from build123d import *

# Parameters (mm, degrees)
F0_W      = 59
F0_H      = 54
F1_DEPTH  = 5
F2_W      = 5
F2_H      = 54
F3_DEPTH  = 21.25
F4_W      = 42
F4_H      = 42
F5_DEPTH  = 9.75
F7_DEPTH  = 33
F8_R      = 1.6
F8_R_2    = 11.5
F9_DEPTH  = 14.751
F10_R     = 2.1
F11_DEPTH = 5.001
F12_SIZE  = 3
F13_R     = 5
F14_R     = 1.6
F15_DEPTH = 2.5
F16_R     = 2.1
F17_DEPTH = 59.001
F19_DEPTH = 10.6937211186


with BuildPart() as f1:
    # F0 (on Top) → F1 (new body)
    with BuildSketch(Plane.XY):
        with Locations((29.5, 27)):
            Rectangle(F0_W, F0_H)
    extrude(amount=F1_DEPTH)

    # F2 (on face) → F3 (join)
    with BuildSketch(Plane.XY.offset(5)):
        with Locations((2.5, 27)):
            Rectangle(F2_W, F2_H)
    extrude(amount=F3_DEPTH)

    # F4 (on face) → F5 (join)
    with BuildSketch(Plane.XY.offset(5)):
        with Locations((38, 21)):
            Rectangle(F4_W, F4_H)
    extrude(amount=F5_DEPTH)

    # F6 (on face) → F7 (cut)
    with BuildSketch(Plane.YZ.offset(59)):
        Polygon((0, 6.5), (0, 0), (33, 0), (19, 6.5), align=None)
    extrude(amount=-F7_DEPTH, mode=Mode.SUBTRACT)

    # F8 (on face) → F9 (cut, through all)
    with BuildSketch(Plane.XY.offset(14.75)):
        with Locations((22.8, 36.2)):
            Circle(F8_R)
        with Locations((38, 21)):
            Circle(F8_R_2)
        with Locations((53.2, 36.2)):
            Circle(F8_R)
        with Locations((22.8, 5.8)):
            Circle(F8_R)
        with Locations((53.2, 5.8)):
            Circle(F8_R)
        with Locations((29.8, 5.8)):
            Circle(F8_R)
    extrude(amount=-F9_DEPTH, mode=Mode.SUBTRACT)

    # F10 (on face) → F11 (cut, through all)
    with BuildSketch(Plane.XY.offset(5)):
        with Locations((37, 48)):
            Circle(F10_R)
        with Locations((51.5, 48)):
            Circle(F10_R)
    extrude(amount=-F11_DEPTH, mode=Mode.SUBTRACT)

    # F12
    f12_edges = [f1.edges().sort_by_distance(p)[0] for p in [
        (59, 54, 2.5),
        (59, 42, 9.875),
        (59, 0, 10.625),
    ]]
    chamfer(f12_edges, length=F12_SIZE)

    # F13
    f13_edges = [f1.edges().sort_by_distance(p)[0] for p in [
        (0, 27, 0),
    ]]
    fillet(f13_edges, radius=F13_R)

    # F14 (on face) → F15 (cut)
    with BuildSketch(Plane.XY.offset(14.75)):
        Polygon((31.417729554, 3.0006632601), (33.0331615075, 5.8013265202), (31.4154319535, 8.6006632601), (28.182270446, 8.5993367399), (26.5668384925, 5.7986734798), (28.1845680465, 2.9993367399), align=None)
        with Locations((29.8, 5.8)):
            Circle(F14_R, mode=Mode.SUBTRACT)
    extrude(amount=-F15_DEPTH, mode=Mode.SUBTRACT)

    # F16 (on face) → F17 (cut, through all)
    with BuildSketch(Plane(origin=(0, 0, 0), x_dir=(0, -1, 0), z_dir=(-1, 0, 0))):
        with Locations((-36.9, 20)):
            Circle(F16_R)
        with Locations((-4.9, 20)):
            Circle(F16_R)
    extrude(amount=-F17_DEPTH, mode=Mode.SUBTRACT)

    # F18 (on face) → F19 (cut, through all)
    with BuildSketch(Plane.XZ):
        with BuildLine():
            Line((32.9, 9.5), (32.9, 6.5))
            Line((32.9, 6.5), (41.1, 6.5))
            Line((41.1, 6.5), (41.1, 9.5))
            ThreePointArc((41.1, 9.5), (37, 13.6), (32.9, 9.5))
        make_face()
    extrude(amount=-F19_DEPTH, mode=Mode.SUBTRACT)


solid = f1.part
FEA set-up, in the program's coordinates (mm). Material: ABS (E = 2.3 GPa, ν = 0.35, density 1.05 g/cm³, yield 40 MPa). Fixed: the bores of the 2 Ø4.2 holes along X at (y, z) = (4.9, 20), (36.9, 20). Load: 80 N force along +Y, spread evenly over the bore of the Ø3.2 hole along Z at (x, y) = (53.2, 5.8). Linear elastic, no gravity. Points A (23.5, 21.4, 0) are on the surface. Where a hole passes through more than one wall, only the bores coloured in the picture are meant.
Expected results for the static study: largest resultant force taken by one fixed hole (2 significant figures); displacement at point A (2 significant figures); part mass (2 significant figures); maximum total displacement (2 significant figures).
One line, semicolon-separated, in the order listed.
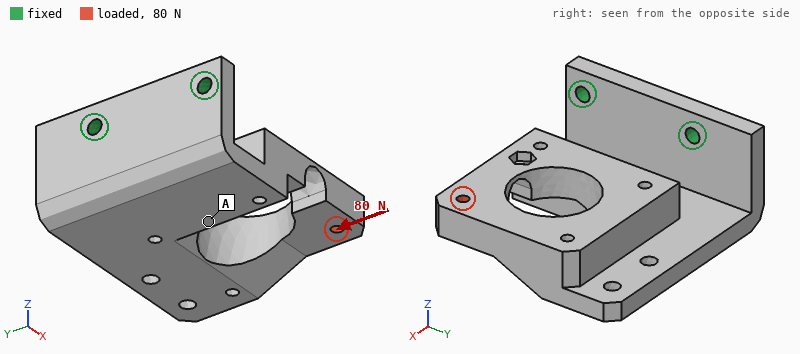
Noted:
120 N; 0.27 mm; 29 g; 0.96 mm
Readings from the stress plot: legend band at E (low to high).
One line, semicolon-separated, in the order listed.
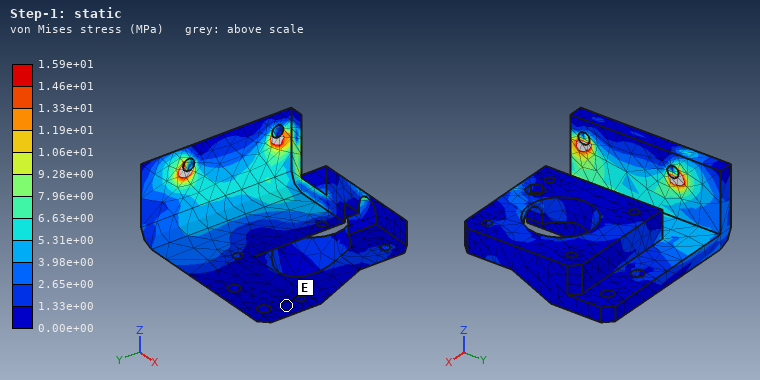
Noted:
0.00e+00 to 1.33e+00 MPa
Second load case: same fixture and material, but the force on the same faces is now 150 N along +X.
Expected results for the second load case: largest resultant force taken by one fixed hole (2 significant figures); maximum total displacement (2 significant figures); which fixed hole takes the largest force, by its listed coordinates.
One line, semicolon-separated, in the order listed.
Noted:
140 N; 0.84 mm; (4.9, 20)
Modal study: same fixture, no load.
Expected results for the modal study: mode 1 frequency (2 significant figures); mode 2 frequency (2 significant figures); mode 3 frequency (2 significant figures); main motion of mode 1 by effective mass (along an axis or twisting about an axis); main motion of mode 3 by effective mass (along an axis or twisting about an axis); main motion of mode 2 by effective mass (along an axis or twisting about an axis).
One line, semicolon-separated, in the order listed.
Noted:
210 Hz; 480 Hz; 970 Hz; along Z; along X; along Y
